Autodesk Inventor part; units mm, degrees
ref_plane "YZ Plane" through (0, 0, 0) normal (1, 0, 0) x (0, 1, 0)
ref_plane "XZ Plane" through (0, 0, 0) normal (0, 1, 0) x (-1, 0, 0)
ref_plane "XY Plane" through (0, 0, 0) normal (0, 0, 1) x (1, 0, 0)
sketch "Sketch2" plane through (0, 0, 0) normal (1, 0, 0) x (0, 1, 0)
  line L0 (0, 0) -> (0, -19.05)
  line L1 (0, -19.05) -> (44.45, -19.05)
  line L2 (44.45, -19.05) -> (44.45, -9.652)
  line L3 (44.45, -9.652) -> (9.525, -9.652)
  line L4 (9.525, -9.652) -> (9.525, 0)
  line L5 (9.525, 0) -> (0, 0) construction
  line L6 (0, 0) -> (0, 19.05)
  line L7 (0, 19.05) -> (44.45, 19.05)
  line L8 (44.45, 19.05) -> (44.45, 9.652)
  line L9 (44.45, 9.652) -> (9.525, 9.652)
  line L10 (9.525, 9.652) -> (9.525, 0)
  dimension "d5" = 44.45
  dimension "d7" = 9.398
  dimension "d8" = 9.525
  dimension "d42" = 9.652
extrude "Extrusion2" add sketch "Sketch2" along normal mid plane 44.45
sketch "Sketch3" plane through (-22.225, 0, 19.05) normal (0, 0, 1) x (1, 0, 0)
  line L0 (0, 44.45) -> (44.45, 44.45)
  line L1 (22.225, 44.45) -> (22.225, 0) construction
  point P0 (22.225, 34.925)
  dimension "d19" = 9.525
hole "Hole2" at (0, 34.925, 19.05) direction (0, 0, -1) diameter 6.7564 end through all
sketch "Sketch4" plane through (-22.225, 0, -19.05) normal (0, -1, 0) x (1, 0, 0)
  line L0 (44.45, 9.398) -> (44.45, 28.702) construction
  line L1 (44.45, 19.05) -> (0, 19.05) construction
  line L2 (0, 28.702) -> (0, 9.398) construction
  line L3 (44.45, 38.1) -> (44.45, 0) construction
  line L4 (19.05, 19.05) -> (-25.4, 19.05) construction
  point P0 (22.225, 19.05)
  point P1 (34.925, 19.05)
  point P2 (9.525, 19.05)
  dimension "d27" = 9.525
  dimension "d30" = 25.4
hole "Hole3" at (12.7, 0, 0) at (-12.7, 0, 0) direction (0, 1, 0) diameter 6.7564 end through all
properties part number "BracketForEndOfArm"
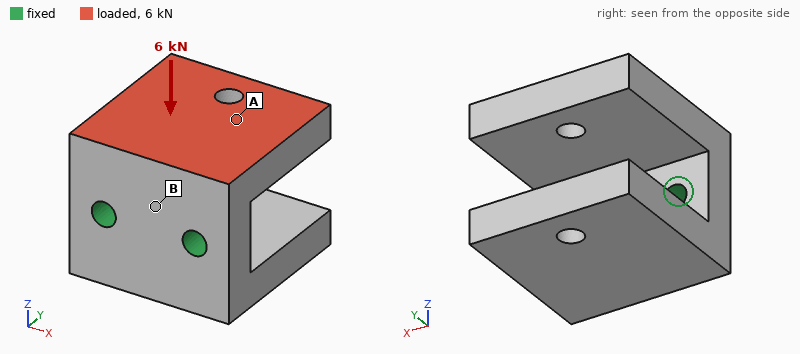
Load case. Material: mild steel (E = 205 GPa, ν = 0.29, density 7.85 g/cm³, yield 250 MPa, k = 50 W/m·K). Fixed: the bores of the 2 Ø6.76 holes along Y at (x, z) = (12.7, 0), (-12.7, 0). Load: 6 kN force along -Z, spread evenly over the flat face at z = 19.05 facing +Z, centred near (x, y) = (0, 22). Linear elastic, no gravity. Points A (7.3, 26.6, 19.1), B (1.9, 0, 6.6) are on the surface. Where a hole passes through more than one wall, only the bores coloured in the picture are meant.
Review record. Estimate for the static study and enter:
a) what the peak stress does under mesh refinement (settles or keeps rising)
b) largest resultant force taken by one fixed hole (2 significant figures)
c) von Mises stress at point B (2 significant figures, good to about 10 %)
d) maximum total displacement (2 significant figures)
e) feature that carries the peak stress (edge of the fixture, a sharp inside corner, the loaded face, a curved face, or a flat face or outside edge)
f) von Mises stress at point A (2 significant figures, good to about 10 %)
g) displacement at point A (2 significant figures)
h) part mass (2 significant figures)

keeps rising
3.1 kN
100 MPa
0.13 mm
edge of the fixture
32 MPa
0.071 mm
350 g
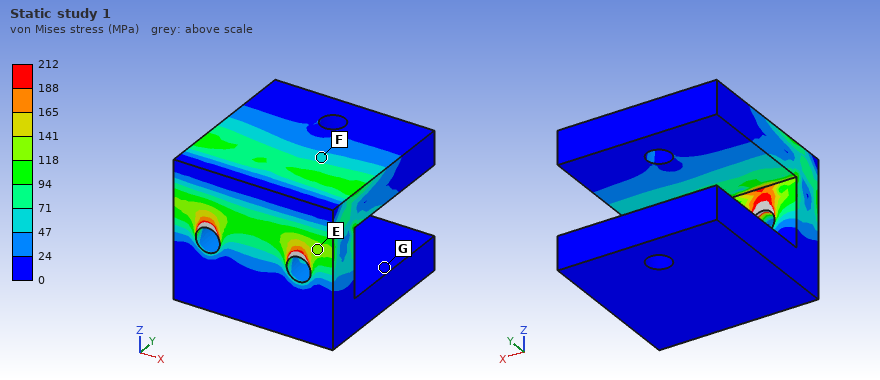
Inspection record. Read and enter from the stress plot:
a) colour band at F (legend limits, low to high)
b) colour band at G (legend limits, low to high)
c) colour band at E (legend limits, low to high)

47 to 71 MPa
0 to 24 MPa
118 to 141 MPa
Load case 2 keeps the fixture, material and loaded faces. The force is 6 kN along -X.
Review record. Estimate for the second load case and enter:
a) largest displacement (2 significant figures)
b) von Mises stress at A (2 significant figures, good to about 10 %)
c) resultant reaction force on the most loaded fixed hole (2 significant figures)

27 µm
23 MPa
5.7 kN
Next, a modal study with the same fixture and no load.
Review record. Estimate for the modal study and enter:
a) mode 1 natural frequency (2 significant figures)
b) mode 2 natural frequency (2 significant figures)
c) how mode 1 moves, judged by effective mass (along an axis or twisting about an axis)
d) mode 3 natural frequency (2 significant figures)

3300 Hz
3500 Hz
along Z
6700 Hz
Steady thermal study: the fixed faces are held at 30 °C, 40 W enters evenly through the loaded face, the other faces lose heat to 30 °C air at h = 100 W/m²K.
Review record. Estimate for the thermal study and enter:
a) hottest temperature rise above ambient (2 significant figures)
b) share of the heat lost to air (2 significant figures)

38 K
28 %
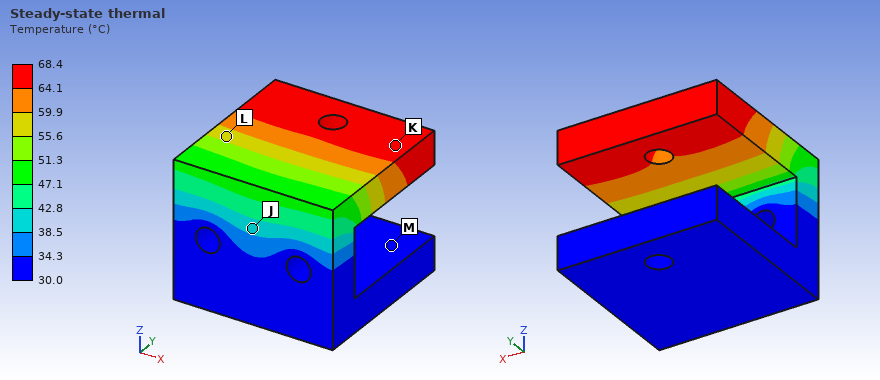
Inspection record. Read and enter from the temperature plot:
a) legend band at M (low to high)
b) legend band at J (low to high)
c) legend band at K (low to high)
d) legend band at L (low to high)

30.0 to 34.3 °C
38.5 to 42.8 °C
64.1 to 68.4 °C
55.6 to 59.9 °C
